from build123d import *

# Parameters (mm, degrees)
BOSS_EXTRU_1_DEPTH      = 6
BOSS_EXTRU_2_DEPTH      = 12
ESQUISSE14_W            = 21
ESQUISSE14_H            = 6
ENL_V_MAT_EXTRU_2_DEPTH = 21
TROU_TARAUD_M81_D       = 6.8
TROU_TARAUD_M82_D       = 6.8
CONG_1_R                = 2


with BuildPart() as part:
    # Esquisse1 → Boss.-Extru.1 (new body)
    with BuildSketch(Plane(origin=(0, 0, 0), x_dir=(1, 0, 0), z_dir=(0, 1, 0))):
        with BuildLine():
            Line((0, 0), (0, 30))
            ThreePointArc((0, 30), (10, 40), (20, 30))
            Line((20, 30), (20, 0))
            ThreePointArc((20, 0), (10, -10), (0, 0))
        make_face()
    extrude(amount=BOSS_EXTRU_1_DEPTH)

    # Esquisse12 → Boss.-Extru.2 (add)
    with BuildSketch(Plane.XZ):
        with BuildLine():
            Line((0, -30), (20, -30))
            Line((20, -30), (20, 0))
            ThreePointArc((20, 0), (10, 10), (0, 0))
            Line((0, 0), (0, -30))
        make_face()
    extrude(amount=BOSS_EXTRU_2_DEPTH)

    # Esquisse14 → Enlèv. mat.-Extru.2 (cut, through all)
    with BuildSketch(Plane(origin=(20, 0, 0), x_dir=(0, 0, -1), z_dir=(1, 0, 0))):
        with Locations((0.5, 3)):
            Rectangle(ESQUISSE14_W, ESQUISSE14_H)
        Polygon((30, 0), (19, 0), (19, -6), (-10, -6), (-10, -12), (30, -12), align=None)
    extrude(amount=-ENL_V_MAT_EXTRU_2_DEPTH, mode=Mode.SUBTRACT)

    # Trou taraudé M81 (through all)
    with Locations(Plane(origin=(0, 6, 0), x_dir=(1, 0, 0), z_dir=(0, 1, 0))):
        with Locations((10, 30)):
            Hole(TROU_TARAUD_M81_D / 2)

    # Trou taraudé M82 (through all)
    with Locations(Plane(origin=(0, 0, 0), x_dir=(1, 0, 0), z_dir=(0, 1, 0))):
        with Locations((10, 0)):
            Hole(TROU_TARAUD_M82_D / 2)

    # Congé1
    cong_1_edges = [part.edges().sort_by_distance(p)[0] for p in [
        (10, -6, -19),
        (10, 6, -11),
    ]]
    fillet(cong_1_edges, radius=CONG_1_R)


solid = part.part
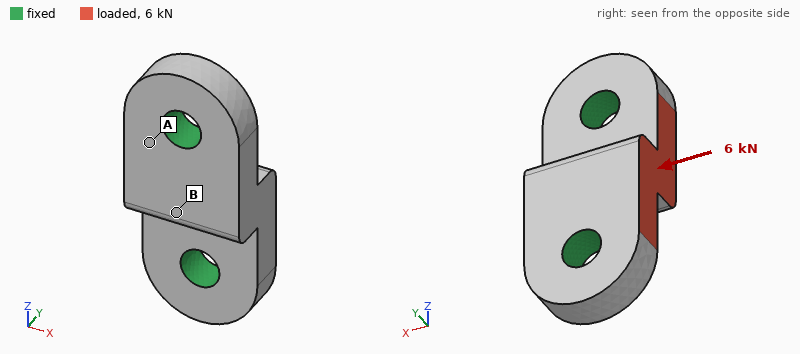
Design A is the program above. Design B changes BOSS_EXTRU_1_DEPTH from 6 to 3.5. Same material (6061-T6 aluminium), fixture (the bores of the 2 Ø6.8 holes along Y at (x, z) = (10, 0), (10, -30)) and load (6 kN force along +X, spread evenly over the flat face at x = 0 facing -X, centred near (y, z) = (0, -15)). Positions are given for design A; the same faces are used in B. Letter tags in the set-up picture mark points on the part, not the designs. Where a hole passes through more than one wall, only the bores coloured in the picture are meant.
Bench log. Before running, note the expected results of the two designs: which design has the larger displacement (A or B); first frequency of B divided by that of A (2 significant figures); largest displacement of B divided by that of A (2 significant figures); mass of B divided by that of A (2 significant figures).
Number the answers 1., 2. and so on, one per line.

1. B
2. 0.88
3. 1.3
4. 0.79
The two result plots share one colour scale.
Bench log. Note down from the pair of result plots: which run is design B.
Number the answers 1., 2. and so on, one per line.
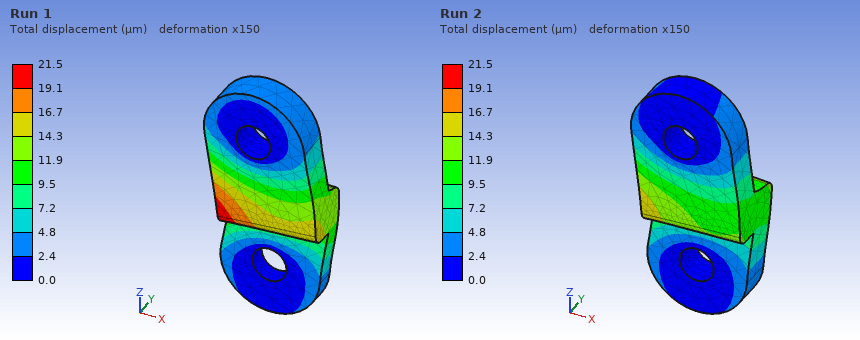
1. Run 1
